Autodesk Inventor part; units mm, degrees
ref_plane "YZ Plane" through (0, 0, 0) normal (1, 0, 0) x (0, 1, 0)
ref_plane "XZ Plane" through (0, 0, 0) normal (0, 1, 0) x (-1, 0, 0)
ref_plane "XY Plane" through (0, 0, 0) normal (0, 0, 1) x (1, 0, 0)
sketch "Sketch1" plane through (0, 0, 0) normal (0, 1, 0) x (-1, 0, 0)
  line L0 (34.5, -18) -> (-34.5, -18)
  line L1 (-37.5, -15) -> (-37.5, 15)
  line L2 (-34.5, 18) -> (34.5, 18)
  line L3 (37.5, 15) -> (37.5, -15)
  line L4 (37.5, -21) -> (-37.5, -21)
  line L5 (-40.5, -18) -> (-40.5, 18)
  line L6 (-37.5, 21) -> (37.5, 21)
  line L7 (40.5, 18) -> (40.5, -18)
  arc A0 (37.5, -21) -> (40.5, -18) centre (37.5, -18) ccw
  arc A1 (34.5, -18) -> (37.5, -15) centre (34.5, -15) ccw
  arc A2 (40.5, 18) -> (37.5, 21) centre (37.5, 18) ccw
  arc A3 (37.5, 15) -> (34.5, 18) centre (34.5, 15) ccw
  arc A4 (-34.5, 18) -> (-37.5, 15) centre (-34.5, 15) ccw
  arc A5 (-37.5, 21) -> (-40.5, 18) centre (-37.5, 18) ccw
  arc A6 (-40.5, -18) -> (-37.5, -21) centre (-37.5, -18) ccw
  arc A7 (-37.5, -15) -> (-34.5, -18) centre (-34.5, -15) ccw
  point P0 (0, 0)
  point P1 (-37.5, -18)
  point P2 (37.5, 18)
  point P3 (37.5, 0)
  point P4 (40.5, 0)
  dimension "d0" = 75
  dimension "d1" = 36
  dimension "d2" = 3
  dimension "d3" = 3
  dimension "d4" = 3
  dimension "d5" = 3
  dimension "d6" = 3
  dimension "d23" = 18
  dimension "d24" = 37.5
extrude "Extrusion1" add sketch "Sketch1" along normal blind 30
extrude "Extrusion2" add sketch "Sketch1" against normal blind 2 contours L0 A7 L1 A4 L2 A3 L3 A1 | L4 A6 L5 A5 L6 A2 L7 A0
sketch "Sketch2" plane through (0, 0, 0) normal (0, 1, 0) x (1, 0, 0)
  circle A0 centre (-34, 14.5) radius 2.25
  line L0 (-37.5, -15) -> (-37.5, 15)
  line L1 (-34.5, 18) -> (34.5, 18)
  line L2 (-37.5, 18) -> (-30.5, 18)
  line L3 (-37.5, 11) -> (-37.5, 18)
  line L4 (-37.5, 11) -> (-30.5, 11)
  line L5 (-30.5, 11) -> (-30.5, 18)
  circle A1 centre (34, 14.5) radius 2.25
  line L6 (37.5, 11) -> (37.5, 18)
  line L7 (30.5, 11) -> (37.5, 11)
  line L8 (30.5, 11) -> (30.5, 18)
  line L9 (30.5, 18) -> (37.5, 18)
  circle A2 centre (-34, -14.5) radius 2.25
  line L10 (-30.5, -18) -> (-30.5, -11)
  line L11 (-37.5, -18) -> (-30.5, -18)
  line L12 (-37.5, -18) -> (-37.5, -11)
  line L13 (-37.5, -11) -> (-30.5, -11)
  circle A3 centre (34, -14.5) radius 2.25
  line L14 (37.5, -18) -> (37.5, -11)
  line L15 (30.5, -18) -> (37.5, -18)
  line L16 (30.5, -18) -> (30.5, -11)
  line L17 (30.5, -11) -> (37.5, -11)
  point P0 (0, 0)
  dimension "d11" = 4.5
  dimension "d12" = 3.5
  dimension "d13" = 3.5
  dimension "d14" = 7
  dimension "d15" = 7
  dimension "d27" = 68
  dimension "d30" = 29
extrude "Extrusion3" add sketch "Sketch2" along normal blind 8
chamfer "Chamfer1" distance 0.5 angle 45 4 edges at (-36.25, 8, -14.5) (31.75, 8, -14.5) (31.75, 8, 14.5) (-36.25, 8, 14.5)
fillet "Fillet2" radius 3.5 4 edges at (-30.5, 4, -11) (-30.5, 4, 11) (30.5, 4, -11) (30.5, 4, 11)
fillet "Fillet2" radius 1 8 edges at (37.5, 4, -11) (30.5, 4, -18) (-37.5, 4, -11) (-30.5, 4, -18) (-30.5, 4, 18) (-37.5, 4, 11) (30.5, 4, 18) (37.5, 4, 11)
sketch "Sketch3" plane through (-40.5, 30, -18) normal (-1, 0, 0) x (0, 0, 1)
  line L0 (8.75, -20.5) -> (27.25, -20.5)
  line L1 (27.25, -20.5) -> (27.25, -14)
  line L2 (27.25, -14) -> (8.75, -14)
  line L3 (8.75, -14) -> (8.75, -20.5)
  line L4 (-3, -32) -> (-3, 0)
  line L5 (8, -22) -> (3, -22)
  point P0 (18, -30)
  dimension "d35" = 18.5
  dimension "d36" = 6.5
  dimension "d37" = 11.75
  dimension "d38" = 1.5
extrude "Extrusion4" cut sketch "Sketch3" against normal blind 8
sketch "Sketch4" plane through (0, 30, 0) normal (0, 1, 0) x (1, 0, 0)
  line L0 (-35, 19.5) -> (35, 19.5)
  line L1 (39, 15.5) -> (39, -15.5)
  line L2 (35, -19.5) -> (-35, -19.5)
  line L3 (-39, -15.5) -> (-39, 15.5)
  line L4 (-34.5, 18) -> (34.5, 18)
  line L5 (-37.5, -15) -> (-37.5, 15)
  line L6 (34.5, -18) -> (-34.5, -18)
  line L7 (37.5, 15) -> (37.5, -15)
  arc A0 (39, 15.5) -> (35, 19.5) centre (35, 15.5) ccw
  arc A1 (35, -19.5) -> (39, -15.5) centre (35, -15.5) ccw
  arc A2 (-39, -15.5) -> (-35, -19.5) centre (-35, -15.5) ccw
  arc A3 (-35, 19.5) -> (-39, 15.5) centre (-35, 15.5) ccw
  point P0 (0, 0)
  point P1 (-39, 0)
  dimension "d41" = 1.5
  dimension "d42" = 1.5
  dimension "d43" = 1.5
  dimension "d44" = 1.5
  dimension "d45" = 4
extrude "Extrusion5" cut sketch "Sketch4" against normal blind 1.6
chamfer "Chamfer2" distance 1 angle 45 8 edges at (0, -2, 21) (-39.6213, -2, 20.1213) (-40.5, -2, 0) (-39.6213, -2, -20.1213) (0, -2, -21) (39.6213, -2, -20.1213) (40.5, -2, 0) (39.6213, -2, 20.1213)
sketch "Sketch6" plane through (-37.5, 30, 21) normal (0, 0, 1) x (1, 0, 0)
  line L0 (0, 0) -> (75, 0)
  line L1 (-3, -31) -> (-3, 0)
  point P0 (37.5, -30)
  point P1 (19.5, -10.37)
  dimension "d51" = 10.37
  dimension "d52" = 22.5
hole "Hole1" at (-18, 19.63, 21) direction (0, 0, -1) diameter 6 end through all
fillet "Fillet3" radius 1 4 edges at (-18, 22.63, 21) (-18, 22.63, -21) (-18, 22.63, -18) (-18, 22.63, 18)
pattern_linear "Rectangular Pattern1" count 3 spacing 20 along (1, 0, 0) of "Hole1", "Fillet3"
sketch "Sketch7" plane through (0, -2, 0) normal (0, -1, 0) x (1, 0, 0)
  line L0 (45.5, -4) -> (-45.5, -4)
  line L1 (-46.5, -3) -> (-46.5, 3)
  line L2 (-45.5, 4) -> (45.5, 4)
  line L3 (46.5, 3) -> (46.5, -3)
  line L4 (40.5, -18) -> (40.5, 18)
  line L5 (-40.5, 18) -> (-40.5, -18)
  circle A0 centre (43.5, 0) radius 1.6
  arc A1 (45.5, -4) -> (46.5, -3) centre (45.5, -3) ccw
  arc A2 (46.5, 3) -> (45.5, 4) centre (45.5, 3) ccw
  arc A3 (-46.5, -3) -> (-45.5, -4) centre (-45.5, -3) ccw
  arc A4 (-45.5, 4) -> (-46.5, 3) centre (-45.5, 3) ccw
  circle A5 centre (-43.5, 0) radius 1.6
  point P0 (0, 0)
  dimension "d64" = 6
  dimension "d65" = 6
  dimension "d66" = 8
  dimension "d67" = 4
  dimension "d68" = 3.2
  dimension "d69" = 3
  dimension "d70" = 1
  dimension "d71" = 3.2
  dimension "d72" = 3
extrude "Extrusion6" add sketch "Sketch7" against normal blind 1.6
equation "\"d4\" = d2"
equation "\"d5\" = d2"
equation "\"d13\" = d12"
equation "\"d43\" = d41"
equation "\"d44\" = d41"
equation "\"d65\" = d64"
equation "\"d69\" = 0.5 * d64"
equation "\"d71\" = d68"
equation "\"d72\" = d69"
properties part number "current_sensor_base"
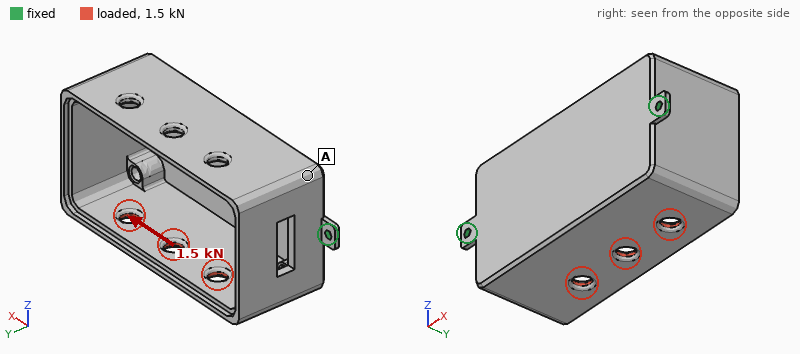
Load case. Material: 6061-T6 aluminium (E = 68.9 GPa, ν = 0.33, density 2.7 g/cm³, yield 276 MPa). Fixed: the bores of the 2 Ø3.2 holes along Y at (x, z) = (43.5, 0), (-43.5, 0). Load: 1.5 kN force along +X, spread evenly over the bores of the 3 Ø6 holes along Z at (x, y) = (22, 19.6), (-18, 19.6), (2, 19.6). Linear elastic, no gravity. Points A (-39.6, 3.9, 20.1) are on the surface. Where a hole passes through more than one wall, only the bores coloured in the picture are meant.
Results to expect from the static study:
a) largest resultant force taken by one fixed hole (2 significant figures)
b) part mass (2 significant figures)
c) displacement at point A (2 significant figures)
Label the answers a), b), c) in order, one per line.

a) 910 N
b) 74 g
c) 0.093 mm
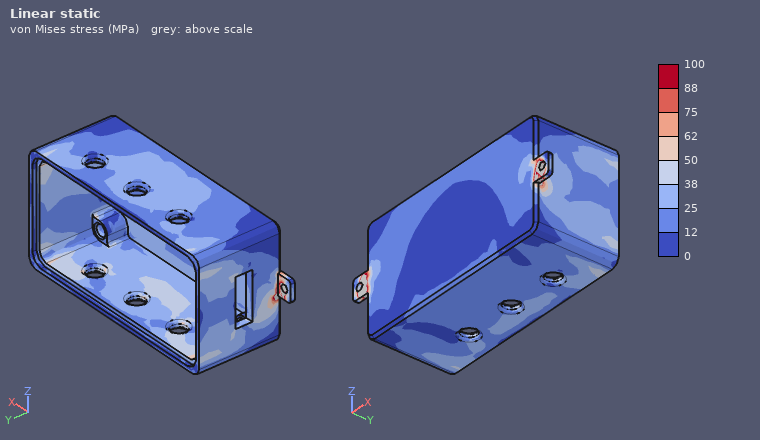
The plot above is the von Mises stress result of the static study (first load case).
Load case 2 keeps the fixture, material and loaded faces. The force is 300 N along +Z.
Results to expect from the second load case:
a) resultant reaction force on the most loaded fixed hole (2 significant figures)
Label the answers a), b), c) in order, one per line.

a) 160 N
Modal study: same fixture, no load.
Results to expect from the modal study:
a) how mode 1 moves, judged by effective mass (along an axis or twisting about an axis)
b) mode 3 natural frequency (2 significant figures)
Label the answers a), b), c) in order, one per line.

a) along Z
b) 3200 Hz
